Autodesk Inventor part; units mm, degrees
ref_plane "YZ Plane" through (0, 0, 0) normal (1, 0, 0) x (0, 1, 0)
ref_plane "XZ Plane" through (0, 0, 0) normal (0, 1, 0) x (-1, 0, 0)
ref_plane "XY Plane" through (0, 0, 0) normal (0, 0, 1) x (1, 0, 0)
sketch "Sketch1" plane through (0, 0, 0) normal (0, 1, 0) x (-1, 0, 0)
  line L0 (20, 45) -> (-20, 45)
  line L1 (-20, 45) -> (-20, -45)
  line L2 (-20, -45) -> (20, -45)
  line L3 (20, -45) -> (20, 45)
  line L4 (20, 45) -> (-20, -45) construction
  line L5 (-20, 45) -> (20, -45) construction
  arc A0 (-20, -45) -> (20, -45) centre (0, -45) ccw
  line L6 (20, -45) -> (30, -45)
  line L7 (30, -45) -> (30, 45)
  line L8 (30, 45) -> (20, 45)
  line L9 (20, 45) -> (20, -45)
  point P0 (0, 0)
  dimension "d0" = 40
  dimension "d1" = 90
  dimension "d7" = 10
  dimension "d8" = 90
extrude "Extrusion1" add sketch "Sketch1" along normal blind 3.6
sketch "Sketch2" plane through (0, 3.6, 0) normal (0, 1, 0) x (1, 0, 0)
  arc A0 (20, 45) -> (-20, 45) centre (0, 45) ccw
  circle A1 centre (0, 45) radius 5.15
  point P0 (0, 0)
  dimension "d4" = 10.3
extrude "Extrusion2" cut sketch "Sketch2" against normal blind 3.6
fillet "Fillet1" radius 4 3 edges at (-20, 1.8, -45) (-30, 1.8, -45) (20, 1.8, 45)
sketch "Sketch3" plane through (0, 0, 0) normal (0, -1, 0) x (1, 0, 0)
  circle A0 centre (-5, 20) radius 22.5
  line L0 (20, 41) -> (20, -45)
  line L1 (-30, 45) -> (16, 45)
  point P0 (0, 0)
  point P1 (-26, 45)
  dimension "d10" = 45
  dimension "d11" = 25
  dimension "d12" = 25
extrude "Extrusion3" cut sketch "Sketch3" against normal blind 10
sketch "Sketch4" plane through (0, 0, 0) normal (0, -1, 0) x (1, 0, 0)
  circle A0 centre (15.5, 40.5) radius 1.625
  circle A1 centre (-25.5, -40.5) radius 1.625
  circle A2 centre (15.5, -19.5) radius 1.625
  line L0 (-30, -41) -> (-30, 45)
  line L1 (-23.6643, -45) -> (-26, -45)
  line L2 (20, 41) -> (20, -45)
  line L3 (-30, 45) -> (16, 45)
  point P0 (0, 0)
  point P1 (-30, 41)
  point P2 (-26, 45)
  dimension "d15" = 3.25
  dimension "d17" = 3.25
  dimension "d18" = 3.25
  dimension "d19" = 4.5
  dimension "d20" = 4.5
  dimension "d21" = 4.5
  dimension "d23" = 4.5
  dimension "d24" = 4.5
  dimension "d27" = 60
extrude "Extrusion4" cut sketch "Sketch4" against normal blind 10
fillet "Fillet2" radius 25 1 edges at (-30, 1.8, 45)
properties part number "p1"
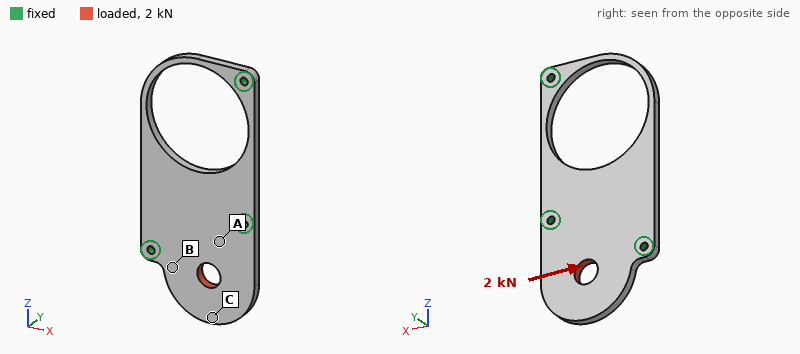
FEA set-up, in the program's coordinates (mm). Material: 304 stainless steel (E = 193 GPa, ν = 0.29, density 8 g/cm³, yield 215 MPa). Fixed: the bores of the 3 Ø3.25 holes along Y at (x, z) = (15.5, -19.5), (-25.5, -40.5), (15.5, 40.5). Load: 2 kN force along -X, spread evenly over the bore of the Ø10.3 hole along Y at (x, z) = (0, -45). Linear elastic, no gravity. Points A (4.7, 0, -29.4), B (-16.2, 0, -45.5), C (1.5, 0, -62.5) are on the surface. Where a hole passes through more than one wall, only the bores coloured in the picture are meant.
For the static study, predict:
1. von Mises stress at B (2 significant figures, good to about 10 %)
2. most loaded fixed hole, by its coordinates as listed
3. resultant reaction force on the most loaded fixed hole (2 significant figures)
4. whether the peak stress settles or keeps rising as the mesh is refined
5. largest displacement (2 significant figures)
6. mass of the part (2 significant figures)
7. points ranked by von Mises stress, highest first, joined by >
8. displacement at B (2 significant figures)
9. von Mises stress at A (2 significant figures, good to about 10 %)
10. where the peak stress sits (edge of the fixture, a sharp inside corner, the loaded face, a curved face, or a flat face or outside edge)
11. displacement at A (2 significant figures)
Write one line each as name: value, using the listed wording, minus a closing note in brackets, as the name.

von Mises stress at B: 34 MPa
most loaded fixed hole, by its coordinates as listed: (-25.5, -40.5)
resultant reaction force on the most loaded fixed hole: 1.4 kN
whether the peak stress settles or keeps rising as the mesh is refined: keeps rising
largest displacement: 5.6 µm
mass of the part: 95 g
points ranked by von Mises stress, highest first, joined by >: B > A > C
displacement at B: 2.2 µm
von Mises stress at A: 11 MPa
where the peak stress sits: edge of the fixture
displacement at A: 1.6 µm
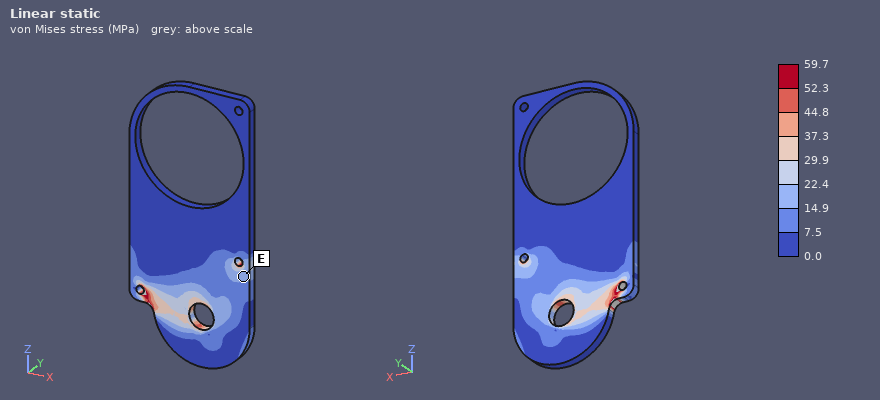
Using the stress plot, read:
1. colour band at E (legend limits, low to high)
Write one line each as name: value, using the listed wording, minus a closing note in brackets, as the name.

colour band at E: 14.9 to 22.4 MPa
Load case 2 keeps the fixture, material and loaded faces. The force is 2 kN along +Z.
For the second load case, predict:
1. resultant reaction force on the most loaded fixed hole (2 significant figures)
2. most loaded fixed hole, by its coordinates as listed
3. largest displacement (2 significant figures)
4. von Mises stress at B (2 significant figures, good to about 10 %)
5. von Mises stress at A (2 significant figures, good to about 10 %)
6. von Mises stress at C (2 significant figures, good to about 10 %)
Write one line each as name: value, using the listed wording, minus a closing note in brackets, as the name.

resultant reaction force on the most loaded fixed hole: 1.2 kN
most loaded fixed hole, by its coordinates as listed: (15.5, -19.5)
largest displacement: 3.9 µm
von Mises stress at B: 8.2 MPa
von Mises stress at A: 15 MPa
von Mises stress at C: 8.7 MPa
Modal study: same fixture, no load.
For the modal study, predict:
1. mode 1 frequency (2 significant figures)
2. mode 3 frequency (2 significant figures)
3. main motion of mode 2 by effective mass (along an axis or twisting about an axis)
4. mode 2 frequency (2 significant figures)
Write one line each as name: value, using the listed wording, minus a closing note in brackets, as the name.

mode 1 frequency: 1700 Hz
mode 3 frequency: 3700 Hz
main motion of mode 2 by effective mass: along Y
mode 2 frequency: 2400 Hz
